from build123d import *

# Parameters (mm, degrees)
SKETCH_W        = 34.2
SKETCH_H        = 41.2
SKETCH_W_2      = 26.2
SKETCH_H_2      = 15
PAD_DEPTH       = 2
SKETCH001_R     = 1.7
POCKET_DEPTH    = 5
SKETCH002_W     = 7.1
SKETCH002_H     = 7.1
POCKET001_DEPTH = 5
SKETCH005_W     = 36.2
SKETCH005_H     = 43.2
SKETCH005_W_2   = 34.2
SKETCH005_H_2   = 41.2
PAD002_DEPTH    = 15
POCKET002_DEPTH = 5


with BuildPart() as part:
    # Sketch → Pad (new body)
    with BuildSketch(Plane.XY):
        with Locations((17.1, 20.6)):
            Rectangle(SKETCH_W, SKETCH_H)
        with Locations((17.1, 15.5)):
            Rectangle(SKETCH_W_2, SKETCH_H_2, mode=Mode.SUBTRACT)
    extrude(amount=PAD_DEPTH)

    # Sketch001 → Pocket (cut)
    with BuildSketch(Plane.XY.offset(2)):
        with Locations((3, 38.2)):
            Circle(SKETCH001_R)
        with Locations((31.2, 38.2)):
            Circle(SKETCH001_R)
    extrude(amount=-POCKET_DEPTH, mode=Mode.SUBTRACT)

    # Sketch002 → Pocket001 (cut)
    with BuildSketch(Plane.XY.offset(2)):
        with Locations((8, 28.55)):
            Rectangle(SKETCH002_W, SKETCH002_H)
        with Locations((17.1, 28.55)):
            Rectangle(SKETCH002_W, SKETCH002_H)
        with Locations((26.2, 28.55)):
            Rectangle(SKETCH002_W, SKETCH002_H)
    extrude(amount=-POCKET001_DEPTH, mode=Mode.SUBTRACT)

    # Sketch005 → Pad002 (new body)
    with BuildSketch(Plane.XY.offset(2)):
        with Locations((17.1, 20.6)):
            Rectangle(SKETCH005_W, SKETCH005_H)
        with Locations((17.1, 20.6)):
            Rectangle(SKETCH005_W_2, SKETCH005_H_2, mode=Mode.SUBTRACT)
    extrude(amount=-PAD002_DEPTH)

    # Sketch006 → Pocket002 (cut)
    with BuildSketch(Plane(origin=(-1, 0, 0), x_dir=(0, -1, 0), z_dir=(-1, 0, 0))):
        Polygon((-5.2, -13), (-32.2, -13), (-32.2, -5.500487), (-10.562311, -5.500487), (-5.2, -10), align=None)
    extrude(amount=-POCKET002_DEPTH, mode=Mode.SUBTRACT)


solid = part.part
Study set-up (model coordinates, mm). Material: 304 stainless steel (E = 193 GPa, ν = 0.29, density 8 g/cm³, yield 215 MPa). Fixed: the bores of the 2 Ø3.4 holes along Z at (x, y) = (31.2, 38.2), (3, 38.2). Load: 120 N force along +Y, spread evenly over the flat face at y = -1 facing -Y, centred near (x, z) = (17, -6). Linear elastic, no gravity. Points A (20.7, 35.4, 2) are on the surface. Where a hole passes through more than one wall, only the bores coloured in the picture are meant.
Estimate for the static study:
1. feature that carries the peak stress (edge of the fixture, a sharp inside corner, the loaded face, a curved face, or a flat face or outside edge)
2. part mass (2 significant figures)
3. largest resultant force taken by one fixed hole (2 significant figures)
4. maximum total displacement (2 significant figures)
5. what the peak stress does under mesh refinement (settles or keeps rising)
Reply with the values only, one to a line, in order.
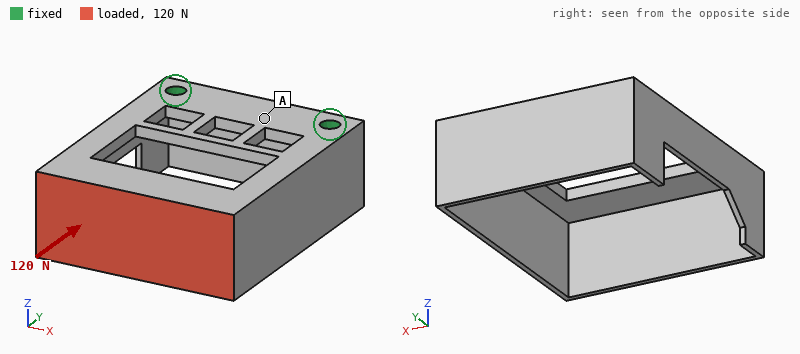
edge of the fixture
31 g
62 N
50 µm
keeps rising
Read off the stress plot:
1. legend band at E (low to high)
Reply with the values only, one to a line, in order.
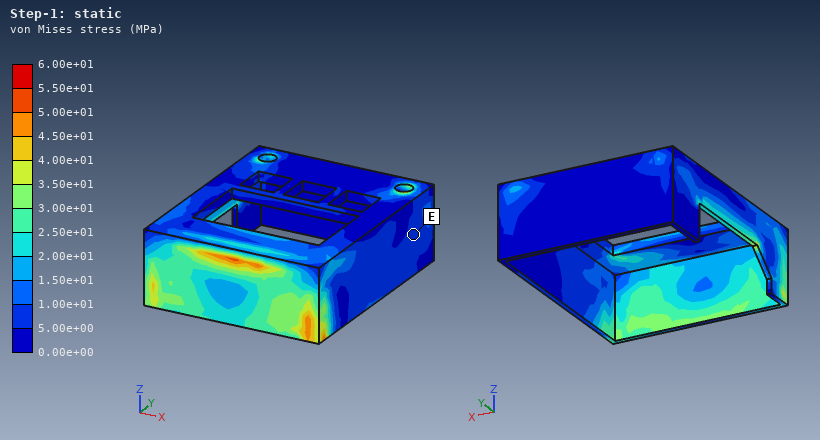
5.00e+00 to 1.00e+01 MPa
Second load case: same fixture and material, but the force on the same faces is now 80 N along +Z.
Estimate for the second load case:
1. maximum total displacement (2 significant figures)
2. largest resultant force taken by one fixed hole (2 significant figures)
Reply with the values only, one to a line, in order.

99 µm
52 N
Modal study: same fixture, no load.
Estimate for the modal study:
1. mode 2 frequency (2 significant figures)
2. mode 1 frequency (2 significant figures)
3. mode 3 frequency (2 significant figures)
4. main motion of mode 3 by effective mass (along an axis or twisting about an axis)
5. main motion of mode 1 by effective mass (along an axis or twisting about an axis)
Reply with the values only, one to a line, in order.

2100 Hz
1600 Hz
3600 Hz
along X
along Z
